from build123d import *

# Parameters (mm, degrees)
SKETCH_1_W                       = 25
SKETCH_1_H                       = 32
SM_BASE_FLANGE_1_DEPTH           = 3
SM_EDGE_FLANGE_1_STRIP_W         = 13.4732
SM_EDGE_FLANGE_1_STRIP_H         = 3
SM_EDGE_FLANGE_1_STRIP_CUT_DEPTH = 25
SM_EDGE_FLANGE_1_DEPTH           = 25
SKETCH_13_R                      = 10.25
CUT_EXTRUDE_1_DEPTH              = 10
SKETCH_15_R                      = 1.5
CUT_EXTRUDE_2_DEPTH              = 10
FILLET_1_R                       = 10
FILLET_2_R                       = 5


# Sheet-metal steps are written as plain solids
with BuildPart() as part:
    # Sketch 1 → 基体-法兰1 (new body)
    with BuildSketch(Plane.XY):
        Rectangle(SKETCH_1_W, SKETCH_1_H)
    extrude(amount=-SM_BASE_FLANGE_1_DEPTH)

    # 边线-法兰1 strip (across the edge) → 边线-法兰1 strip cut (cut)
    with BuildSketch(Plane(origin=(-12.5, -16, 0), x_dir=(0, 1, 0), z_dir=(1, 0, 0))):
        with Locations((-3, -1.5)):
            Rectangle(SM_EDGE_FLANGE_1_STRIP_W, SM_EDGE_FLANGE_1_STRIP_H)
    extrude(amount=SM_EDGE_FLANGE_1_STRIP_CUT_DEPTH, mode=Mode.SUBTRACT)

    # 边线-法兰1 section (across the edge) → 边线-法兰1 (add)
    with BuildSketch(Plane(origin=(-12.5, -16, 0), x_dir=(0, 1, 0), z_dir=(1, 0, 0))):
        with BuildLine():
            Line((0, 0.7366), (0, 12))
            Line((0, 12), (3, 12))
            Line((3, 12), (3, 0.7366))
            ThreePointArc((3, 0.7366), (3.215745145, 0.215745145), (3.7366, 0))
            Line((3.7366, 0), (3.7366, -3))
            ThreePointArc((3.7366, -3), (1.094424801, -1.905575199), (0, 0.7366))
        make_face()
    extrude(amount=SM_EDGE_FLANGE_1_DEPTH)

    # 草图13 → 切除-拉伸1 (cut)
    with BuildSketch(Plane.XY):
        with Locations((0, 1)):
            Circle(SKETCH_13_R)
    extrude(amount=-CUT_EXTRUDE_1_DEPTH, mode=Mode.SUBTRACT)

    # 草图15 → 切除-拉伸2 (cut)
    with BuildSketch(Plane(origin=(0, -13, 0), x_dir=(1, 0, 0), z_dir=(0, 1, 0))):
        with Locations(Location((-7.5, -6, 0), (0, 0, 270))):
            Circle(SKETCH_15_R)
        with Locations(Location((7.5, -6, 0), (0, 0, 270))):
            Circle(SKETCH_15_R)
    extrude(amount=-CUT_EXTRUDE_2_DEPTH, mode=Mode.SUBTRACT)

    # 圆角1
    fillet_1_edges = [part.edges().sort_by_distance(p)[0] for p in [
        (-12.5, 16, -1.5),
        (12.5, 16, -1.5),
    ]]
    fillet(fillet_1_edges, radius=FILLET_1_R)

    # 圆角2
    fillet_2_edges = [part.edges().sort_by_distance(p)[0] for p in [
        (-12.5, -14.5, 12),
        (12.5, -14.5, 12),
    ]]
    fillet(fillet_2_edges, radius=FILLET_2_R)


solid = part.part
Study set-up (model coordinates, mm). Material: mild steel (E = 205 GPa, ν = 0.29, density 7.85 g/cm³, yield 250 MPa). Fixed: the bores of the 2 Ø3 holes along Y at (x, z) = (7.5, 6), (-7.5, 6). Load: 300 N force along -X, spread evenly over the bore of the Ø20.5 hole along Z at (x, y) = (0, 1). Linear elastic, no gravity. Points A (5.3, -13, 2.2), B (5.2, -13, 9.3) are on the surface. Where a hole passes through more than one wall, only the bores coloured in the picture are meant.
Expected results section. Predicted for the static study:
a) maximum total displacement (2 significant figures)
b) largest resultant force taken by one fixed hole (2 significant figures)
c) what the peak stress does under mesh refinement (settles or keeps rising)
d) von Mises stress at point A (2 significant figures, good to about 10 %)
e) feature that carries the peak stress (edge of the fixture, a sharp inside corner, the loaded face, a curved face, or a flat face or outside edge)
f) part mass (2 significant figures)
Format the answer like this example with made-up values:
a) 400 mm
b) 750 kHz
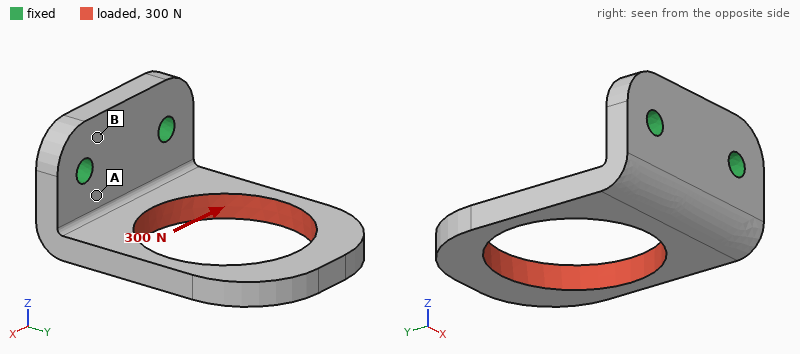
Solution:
a) 38 µm
b) 320 N
c) keeps rising
d) 45 MPa
e) edge of the fixture
f) 16 g
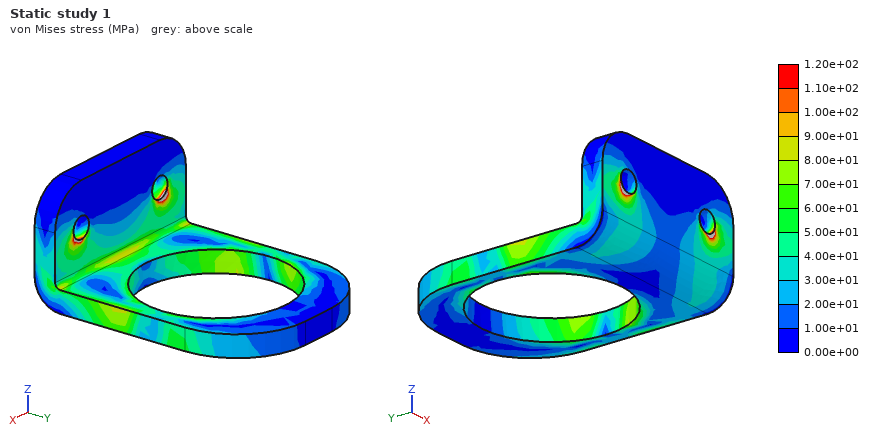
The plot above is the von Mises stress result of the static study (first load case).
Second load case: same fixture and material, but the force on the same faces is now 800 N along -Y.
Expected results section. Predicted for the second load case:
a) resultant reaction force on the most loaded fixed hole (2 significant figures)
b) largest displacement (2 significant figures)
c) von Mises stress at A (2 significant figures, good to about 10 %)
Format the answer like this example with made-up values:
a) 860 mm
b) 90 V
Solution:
a) 400 N
b) 62 µm
c) 73 MPa
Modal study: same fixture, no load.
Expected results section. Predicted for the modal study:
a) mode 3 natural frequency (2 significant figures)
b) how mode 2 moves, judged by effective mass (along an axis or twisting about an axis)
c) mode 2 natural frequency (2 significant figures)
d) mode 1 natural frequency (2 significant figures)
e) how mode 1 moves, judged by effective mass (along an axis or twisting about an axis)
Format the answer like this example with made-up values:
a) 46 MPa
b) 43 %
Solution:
a) 6500 Hz
b) along X
c) 5200 Hz
d) 2000 Hz
e) along Z
